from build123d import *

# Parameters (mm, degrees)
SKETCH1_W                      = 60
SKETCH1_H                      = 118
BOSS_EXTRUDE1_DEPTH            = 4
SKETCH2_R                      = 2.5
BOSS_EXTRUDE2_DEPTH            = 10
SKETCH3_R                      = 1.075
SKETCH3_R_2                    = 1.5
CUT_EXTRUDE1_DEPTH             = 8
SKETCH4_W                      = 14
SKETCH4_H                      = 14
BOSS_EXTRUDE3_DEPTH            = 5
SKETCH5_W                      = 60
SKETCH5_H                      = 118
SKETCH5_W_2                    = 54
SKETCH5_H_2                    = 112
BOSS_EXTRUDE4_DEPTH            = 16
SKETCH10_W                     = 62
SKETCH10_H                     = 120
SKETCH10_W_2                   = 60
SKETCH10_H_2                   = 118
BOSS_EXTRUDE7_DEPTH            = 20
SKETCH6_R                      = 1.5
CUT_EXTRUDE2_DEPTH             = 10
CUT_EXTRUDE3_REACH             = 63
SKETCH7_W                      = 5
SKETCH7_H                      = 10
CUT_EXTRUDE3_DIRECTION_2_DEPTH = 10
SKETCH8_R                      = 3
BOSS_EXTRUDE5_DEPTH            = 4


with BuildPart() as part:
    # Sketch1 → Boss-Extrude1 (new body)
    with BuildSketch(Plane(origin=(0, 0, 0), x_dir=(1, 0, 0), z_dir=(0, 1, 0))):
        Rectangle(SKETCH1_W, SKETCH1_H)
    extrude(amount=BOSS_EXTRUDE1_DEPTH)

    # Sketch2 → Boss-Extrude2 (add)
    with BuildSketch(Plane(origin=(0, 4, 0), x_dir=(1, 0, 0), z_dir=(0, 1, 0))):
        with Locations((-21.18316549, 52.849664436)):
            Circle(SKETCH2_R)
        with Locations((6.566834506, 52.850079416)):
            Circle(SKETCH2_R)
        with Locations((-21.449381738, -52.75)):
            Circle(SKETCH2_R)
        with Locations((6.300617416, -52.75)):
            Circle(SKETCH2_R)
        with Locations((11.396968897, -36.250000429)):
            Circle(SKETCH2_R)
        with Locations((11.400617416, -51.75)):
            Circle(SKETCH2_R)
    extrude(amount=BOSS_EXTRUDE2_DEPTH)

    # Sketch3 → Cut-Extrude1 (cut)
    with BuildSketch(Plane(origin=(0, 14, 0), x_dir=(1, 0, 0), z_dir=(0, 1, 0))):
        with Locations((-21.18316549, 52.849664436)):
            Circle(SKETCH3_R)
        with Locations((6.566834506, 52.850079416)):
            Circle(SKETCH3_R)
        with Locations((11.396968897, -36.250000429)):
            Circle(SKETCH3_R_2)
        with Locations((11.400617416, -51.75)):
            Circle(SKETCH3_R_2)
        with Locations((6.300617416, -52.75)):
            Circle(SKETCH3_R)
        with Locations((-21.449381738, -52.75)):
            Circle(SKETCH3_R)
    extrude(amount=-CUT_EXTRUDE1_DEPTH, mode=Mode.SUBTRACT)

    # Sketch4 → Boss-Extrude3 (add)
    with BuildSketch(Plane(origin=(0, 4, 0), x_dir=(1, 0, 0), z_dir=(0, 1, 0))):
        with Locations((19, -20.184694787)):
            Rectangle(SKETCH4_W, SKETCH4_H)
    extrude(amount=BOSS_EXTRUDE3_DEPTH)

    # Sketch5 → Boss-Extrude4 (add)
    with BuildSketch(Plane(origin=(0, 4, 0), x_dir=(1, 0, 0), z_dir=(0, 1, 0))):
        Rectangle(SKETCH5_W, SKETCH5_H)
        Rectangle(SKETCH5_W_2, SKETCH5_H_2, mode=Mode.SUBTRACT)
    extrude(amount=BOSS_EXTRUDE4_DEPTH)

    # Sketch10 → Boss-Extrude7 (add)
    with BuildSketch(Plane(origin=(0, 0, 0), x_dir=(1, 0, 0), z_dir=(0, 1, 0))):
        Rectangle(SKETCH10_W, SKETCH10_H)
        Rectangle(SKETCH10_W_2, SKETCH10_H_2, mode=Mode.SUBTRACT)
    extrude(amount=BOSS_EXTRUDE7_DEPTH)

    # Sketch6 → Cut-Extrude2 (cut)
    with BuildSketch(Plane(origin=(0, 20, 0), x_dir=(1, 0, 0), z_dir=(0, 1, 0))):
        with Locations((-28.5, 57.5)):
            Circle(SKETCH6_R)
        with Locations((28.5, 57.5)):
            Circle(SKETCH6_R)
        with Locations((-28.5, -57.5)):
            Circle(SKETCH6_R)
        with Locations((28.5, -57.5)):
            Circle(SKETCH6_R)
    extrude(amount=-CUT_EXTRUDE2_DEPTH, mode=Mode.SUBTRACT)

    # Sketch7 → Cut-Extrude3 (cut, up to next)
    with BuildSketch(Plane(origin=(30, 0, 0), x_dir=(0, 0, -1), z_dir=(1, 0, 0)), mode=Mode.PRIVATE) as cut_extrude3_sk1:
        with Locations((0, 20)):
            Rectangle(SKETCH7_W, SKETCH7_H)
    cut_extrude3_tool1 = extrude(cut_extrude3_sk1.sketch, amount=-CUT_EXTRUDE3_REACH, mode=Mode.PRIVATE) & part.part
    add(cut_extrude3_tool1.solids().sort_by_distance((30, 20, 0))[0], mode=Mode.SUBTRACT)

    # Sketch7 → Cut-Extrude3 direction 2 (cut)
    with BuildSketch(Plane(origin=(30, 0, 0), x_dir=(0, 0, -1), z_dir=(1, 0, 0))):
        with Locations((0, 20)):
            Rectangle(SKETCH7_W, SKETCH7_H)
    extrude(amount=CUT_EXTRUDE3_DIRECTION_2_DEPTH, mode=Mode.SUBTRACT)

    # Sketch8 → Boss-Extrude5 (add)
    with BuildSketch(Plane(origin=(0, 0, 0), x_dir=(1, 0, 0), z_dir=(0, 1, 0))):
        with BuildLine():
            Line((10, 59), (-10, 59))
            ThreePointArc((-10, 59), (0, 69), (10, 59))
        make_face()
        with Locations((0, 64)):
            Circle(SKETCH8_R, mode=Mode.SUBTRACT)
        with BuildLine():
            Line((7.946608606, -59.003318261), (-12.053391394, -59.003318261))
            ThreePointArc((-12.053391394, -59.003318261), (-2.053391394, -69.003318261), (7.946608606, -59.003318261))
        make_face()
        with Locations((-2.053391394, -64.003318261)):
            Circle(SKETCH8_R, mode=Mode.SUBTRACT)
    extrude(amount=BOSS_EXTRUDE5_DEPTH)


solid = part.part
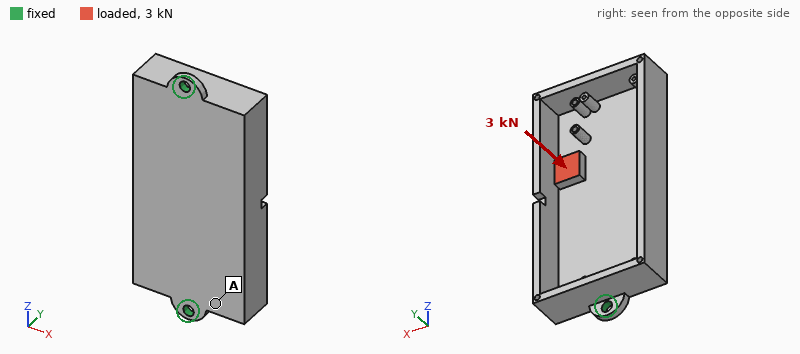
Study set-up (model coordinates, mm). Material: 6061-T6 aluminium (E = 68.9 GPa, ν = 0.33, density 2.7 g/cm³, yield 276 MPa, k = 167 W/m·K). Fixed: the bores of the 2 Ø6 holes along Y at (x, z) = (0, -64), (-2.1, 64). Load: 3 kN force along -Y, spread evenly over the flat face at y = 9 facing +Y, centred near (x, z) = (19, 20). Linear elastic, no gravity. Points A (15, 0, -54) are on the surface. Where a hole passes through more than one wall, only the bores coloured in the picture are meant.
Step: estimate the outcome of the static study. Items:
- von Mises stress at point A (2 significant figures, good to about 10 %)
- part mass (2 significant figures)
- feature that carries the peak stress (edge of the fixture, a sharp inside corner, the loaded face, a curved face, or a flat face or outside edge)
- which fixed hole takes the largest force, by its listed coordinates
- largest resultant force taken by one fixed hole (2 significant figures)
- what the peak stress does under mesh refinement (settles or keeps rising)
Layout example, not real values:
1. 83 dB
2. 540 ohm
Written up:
1. 33 MPa
2. 150 g
3. edge of the fixture
4. (-2.1, 64)
5. 2.2 kN
6. keeps rising
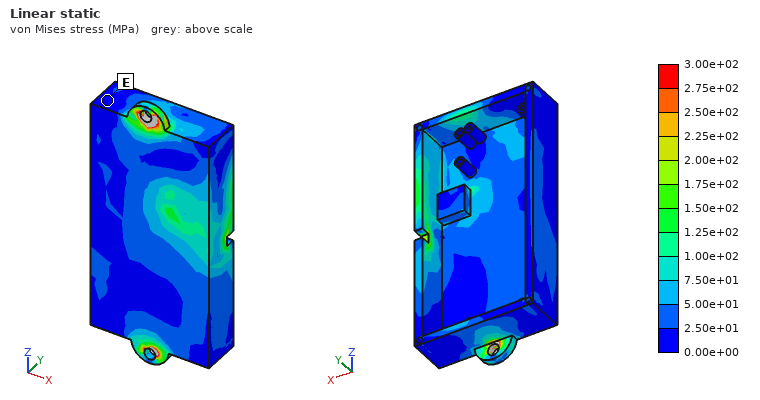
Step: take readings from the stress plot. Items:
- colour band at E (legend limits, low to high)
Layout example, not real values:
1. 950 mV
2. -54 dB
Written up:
1. 0.00e+00 to 2.50e+01 MPa
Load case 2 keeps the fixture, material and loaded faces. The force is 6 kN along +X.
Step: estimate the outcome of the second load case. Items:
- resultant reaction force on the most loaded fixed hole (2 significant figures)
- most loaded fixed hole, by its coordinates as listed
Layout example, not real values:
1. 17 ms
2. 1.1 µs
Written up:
1. 4.0 kN
2. (-2.1, 64)
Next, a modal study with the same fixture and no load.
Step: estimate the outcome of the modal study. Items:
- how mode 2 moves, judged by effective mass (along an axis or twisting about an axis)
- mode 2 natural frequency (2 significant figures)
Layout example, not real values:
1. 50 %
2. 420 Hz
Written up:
1. along Y
2. 2200 Hz
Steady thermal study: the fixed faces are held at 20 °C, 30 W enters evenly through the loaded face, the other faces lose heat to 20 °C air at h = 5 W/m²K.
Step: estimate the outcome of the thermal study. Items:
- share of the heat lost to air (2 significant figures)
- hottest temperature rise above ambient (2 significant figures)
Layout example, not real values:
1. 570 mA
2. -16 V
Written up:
1. 6.8 %
2. 35 K
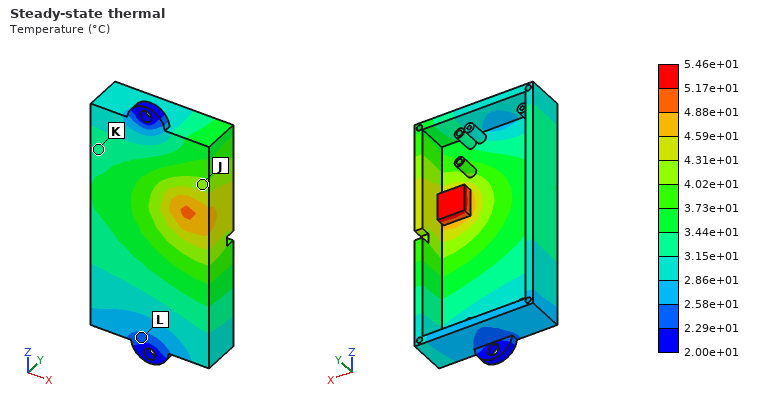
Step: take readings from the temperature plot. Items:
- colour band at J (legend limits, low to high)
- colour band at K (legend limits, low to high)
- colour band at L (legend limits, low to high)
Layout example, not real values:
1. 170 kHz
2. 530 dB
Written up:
1. 4.02e+01 to 4.31e+01 °C
2. 3.15e+01 to 3.44e+01 °C
3. 2.29e+01 to 2.58e+01 °C
